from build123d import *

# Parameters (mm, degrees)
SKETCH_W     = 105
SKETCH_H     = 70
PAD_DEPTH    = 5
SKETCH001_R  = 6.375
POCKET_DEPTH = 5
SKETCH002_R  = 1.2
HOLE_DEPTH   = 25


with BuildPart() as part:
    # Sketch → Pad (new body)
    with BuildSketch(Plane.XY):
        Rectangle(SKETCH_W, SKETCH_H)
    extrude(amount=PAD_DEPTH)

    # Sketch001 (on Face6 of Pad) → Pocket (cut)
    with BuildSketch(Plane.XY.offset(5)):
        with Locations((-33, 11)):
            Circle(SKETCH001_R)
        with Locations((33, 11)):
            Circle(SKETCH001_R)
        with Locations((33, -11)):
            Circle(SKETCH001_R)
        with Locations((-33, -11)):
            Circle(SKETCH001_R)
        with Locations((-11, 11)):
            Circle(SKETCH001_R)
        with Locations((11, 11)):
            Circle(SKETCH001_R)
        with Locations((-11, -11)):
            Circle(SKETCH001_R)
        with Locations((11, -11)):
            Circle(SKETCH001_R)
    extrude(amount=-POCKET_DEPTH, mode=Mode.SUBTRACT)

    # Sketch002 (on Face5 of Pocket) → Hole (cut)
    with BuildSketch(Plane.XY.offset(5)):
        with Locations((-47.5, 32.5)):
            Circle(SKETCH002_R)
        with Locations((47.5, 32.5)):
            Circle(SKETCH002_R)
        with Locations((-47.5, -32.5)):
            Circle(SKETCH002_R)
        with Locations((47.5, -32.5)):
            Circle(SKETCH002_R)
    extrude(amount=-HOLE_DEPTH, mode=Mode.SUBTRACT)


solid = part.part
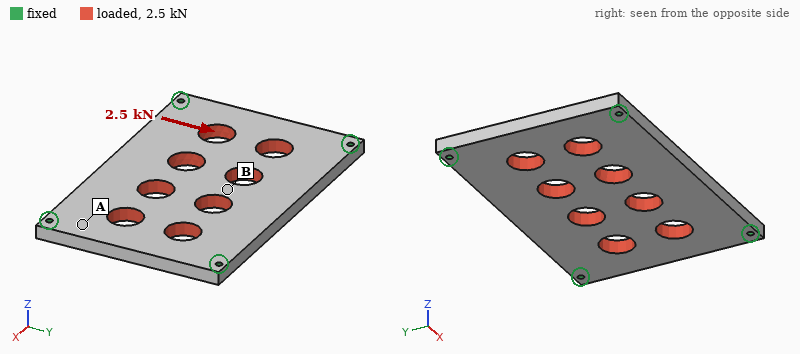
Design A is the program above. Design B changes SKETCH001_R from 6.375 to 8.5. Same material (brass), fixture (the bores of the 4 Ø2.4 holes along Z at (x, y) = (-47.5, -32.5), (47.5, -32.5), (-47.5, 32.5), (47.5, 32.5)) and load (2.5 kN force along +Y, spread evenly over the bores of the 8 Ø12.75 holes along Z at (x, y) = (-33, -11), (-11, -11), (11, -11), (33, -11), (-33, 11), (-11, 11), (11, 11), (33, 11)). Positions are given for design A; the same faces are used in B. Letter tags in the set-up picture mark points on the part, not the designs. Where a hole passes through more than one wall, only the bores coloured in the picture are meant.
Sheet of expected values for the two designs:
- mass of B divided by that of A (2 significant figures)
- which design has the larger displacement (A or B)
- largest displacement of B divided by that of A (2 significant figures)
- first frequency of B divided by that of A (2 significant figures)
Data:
0.87
B
1.7
1.0
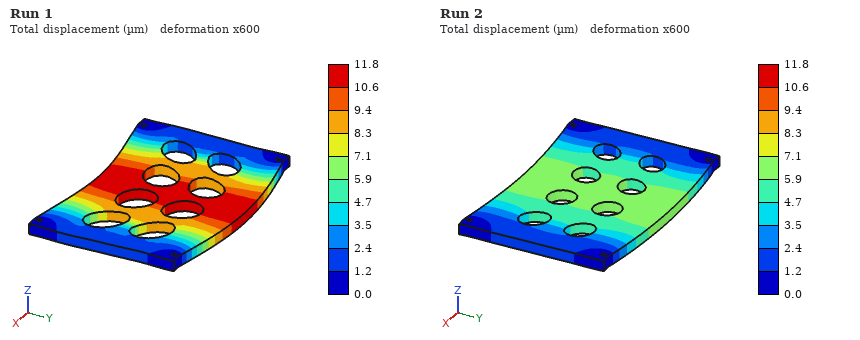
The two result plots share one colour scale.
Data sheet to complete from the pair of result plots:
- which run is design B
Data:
Run 1
